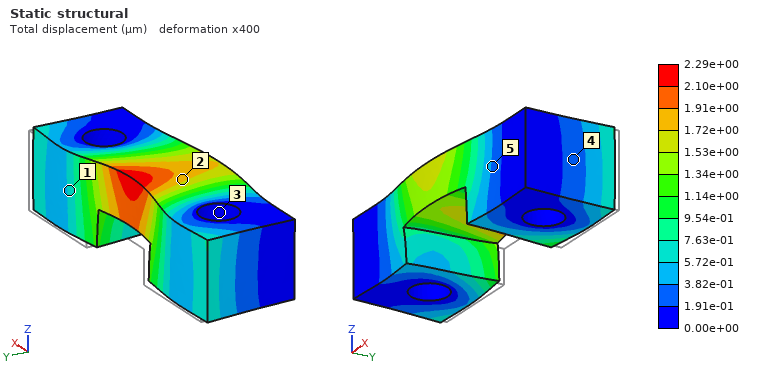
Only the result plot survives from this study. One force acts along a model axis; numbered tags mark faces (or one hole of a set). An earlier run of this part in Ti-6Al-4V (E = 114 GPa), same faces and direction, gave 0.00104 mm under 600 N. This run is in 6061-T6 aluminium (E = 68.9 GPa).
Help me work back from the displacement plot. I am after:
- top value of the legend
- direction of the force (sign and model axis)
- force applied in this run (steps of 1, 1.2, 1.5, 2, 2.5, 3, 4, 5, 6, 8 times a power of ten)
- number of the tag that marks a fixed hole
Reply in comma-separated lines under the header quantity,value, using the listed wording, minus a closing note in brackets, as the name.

quantity,value
top value of the legend,2.29e+00 µm
direction of the force,-Y
force applied in this run,800 N
number of the tag that marks a fixed hole,3
